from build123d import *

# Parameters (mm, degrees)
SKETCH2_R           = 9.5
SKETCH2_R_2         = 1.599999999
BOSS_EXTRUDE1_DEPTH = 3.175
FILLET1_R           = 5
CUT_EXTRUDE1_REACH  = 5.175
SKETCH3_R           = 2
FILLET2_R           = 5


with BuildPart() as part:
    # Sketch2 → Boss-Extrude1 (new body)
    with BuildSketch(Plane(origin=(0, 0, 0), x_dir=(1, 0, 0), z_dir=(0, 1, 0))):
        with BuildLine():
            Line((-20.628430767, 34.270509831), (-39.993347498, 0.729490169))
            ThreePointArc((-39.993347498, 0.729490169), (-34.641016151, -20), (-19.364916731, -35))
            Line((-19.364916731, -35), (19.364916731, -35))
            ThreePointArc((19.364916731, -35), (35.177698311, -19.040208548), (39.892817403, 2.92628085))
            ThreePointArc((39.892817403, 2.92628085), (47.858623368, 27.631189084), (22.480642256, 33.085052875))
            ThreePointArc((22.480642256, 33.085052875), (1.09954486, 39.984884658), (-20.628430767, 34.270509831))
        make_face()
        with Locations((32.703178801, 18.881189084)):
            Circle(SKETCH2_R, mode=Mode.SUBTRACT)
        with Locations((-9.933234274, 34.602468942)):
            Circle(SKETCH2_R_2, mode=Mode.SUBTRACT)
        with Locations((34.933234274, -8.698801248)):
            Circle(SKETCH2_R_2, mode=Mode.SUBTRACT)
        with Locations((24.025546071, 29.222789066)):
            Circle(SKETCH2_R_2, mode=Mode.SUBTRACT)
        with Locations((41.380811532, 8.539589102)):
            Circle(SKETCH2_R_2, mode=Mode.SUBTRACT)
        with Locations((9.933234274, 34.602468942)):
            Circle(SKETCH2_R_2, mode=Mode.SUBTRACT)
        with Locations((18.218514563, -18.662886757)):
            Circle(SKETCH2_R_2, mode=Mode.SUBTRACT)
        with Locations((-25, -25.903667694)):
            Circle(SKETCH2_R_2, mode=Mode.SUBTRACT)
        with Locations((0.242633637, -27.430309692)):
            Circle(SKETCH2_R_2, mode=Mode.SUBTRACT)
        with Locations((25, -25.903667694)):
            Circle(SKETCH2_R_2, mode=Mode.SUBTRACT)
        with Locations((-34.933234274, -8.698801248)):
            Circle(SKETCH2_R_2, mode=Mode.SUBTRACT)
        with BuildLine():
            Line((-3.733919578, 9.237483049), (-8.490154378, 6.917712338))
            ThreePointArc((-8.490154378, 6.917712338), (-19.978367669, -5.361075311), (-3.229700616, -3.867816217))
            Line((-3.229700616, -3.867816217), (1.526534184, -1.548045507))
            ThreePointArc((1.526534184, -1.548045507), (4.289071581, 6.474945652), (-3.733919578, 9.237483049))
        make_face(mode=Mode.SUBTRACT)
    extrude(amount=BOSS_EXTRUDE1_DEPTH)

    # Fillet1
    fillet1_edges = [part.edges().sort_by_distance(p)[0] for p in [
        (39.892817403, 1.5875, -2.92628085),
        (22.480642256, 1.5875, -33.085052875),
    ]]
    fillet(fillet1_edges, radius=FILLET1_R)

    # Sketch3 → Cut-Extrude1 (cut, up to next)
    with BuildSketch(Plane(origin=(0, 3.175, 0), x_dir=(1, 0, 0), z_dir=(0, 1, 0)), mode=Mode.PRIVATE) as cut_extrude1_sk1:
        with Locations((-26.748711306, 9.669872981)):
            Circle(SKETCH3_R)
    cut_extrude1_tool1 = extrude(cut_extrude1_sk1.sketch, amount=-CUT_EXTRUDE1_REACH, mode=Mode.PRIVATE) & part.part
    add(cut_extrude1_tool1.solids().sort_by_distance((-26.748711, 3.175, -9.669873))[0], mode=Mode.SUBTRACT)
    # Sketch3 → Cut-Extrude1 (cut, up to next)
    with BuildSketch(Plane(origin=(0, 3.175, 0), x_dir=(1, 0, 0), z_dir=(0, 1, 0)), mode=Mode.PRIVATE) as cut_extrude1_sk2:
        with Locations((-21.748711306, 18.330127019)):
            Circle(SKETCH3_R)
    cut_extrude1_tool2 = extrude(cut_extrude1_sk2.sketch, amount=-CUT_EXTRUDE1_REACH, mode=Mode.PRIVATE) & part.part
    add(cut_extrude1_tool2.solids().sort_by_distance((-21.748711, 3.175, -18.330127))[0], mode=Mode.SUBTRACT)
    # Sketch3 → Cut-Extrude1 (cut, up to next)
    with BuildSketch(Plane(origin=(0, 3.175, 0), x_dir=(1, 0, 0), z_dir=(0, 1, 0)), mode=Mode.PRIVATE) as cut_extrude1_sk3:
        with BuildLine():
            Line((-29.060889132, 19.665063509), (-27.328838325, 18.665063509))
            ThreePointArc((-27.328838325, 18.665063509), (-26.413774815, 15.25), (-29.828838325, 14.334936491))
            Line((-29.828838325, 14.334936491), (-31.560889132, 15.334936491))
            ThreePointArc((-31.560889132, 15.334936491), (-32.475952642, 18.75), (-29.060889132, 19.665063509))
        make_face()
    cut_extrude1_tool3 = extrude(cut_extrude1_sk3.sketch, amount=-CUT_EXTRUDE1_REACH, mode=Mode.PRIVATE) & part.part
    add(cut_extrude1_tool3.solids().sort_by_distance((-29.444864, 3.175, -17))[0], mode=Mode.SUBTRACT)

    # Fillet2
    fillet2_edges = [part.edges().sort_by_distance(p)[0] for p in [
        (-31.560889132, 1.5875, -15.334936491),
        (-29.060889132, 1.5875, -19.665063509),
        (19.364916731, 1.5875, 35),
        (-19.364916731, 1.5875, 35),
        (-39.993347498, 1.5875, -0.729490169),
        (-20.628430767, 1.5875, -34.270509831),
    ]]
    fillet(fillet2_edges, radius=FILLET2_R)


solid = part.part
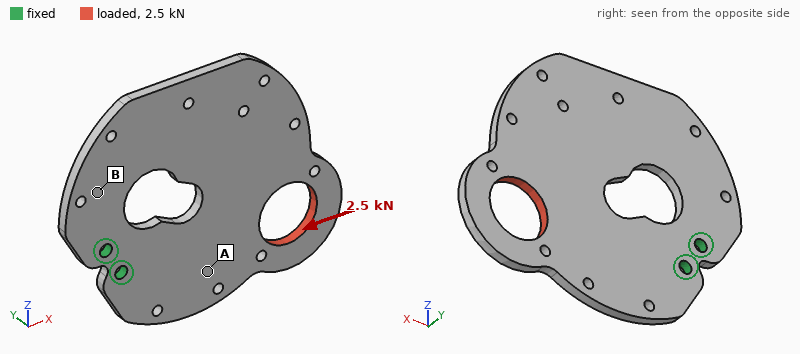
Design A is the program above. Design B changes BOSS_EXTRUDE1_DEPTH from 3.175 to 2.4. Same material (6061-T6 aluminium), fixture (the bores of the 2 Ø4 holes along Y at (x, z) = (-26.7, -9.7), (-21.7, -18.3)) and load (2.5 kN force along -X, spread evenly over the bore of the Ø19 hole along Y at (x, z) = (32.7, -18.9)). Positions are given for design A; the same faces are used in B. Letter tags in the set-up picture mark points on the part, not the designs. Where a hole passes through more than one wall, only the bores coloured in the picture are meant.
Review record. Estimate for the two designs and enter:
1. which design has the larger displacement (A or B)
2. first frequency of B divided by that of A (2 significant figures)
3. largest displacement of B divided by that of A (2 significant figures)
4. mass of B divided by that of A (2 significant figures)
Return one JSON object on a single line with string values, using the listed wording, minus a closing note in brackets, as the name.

{"which design has the larger displacement": "B", "first frequency of B divided by that of A": "0.77", "largest displacement of B divided by that of A": "1.3", "mass of B divided by that of A": "0.76"}
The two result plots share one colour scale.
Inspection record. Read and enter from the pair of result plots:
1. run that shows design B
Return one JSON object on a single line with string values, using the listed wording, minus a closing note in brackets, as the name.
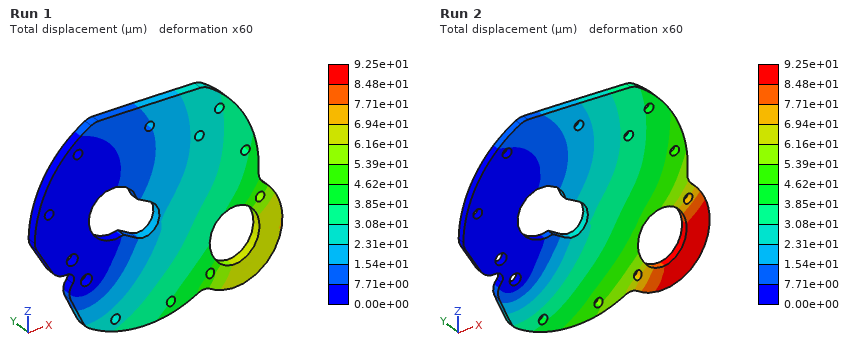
{"run that shows design B": "Run 2"}
